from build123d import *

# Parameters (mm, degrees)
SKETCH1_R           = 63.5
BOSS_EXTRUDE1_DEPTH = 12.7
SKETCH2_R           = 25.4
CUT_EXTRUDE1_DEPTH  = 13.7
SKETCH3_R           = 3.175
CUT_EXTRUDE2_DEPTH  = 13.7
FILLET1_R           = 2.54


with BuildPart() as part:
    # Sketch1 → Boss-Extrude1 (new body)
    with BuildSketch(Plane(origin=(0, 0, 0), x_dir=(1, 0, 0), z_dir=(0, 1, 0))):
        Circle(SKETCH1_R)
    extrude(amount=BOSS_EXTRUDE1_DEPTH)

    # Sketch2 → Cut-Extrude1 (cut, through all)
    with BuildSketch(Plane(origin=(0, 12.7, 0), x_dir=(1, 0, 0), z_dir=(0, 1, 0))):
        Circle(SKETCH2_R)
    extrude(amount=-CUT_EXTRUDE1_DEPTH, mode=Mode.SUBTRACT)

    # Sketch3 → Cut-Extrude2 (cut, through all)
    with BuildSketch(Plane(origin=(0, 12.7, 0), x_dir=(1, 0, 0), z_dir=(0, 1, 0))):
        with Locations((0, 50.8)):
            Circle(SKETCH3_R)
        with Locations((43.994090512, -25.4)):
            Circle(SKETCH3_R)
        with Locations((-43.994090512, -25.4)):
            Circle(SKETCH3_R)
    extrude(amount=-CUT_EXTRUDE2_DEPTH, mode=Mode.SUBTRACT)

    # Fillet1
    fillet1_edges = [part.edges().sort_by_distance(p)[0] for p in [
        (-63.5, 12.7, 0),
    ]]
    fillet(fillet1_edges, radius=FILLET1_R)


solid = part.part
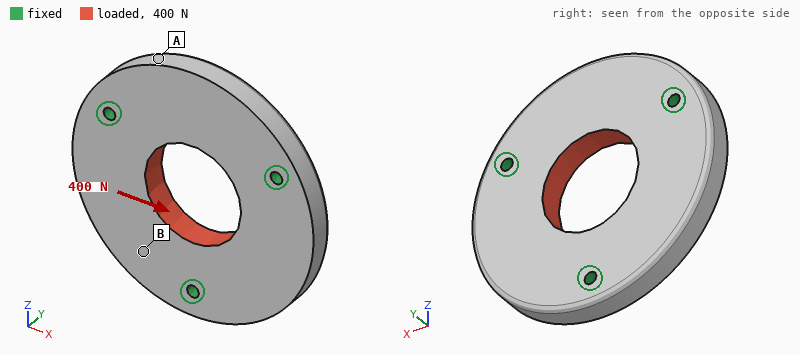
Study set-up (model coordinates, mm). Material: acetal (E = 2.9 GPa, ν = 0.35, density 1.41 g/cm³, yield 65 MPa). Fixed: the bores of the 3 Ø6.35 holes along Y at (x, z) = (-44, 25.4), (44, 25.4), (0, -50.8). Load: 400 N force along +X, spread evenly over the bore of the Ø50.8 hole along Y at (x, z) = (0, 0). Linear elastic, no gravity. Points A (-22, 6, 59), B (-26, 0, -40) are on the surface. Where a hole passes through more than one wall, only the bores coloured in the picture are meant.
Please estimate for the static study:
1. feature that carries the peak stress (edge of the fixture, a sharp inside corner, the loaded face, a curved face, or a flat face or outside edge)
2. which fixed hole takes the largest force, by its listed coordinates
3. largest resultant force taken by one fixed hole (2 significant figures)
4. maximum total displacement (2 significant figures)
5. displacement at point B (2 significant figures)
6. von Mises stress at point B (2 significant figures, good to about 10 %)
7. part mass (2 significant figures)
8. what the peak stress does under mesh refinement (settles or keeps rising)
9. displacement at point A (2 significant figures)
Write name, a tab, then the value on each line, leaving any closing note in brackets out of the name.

feature that carries the peak stress	edge of the fixture
which fixed hole takes the largest force, by its listed coordinates	(0, -50.8)
largest resultant force taken by one fixed hole	150 N
maximum total displacement	7.3 µm
displacement at point B	4.5 µm
von Mises stress at point B	0.21 MPa
part mass	190 g
what the peak stress does under mesh refinement	keeps rising
displacement at point A	1.8 µm
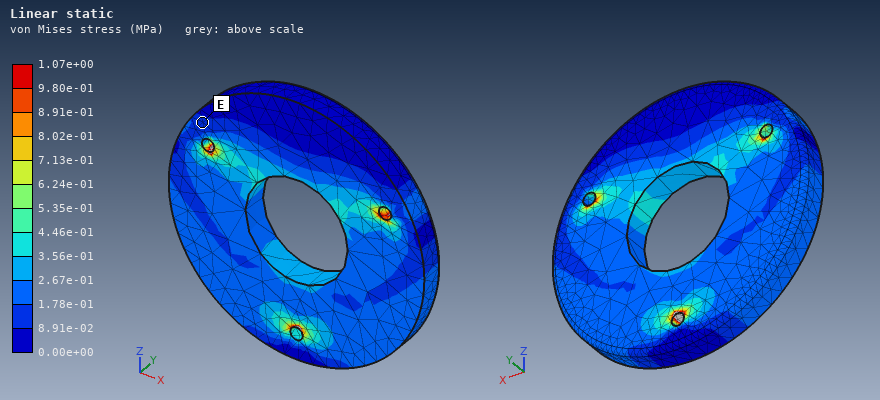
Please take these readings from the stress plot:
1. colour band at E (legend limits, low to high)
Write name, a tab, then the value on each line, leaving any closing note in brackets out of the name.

colour band at E	8.91e-02 to 1.78e-01 MPa
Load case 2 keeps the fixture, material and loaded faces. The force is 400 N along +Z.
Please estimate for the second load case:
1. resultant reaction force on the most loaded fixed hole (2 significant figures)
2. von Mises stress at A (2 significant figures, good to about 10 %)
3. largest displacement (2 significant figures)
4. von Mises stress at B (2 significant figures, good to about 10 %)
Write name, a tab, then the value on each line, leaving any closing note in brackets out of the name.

resultant reaction force on the most loaded fixed hole	140 N
von Mises stress at A	0.25 MPa
largest displacement	8.1 µm
von Mises stress at B	0.11 MPa
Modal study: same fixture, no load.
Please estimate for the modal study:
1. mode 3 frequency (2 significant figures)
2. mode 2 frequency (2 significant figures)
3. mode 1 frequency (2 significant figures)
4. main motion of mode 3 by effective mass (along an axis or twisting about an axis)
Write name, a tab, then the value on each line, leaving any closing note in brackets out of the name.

mode 3 frequency	1500 Hz
mode 2 frequency	1300 Hz
mode 1 frequency	1300 Hz
main motion of mode 3 by effective mass	along Y
